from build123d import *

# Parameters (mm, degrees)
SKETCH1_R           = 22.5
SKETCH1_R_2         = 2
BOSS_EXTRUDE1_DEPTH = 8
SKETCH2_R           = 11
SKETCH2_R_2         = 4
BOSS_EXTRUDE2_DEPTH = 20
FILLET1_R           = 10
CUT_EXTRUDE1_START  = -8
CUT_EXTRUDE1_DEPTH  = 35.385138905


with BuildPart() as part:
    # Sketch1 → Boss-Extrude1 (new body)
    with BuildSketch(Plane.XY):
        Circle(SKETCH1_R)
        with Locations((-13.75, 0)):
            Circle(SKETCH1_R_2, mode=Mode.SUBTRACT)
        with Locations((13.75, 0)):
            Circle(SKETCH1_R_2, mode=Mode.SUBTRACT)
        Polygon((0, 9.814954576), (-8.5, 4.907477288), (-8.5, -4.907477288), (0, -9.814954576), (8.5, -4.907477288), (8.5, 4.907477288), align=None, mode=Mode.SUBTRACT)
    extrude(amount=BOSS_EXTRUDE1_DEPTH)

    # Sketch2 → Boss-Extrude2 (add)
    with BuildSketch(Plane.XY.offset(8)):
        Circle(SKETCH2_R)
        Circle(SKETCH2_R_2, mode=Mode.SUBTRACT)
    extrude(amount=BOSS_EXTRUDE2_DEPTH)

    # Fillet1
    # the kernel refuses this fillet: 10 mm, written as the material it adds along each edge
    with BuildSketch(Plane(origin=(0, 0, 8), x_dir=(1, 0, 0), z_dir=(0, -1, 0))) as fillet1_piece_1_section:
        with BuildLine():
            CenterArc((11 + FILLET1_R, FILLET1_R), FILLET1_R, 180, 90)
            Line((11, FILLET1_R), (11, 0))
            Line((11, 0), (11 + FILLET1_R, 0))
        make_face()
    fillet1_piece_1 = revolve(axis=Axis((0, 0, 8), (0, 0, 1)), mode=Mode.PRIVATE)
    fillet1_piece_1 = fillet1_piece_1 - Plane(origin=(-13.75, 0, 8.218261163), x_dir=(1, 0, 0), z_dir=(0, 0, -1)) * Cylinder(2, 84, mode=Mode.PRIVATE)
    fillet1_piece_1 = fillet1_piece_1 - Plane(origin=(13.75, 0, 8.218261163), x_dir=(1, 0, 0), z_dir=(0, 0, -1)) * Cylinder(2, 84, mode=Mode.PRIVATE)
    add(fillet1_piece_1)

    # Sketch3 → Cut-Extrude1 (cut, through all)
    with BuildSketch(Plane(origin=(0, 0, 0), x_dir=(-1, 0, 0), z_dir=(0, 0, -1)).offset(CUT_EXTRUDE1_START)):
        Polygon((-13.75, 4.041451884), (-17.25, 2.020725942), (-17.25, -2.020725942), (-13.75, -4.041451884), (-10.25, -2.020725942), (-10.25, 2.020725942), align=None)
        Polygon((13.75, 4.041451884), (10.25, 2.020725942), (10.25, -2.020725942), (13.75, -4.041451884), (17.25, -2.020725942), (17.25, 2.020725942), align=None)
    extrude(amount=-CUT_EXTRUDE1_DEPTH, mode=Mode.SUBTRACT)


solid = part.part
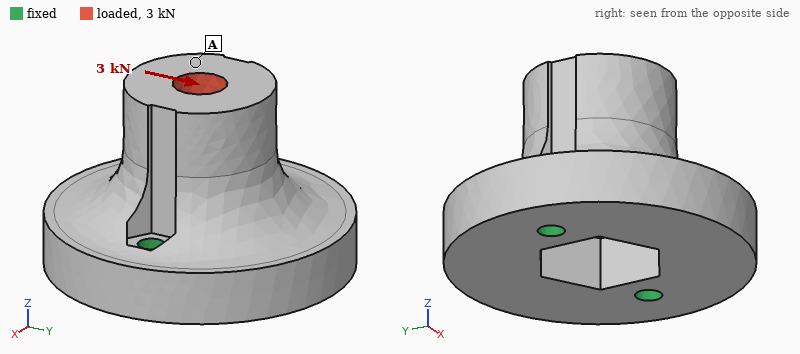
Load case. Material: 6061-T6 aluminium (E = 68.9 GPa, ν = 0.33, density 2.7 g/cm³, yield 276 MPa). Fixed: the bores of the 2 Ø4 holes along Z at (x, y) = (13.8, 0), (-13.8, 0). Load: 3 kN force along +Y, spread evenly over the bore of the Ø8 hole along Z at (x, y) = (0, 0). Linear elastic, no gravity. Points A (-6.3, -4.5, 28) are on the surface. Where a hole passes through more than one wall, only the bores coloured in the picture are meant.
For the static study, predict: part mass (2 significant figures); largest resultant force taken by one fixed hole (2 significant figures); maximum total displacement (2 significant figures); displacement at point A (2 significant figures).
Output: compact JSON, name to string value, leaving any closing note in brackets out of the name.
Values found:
{"part mass": "50 g", "largest resultant force taken by one fixed hole": "1.5 kN", "maximum total displacement": "48 µm", "displacement at point A": "45 µm"}
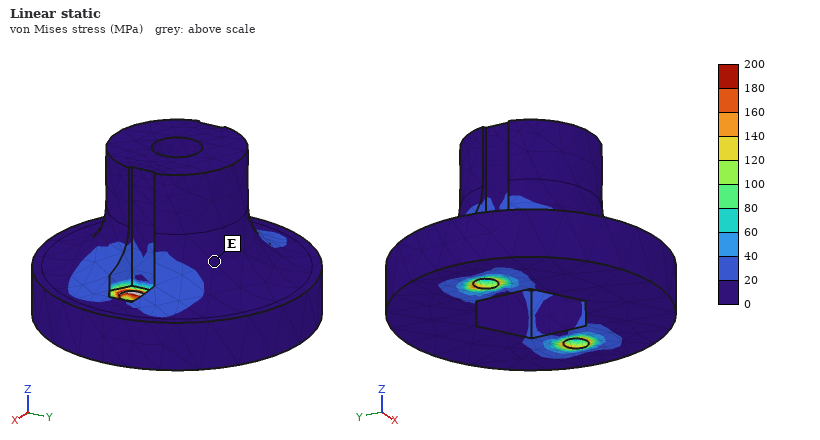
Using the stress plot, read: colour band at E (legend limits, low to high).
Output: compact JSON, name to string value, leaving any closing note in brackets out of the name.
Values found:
{"colour band at E": "0 to 20 MPa"}
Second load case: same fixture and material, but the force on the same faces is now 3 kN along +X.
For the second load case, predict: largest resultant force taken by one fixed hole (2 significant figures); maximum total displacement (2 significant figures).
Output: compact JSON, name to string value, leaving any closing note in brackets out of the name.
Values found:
{"largest resultant force taken by one fixed hole": "2.0 kN", "maximum total displacement": "12 µm"}
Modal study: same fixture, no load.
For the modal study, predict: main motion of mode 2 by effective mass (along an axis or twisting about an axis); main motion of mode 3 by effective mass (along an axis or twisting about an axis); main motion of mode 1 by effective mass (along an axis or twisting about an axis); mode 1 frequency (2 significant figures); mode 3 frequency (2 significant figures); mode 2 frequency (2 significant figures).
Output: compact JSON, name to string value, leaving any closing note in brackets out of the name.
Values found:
{"main motion of mode 2 by effective mass": "along Z", "main motion of mode 3 by effective mass": "along X", "main motion of mode 1 by effective mass": "along Y", "mode 1 frequency": "8300 Hz", "mode 3 frequency": "20 kHz", "mode 2 frequency": "18 kHz"}
